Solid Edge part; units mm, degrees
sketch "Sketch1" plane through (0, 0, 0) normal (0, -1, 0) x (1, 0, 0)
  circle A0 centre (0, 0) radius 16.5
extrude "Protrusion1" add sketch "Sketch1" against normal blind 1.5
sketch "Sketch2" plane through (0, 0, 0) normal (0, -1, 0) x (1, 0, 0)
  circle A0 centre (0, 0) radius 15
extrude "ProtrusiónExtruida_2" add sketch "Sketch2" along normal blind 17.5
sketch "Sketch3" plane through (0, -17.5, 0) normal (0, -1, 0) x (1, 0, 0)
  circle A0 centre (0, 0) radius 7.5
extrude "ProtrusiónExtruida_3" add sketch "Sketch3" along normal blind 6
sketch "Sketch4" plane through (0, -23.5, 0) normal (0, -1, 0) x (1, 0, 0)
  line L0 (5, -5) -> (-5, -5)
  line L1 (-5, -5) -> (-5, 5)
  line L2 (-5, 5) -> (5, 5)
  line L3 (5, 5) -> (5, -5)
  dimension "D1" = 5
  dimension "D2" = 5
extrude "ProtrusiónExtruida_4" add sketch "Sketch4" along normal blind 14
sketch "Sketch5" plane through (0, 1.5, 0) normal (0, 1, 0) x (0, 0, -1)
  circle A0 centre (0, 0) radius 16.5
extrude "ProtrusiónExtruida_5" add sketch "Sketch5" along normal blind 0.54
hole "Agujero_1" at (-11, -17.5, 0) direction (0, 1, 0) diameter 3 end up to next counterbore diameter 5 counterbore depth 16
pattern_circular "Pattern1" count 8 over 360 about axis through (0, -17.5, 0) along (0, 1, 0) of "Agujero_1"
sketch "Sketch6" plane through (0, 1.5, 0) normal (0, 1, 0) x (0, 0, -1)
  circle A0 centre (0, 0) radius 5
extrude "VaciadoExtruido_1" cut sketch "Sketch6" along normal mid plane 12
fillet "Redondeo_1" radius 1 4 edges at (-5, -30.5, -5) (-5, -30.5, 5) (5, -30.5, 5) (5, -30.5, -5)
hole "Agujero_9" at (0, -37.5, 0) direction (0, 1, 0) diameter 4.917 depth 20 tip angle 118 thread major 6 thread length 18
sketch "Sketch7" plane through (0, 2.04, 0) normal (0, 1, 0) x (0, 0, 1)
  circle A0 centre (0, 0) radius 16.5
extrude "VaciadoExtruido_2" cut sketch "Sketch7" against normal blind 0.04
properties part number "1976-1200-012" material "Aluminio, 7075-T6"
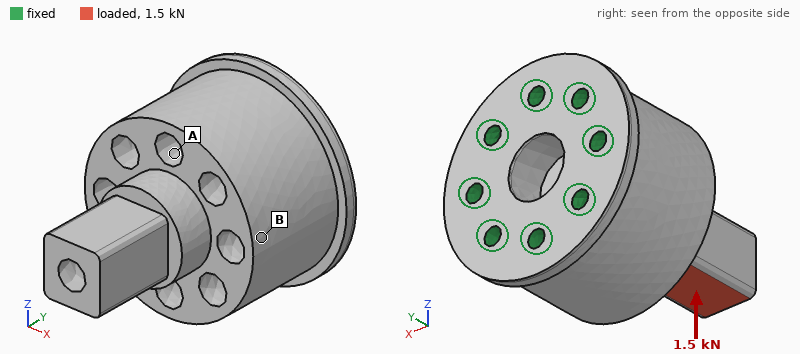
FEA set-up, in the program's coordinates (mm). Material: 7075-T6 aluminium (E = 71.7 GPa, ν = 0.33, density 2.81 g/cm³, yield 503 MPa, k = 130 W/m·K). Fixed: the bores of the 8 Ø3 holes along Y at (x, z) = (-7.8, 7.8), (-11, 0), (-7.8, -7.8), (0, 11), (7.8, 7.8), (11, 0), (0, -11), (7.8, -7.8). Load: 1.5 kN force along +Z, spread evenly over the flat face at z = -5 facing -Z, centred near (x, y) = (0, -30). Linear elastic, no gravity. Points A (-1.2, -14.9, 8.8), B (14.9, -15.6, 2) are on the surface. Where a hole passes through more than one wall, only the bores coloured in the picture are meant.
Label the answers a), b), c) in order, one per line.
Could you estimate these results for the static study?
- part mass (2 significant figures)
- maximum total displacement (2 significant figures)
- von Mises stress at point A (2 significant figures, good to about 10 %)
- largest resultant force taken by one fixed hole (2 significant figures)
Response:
a) 36 g
b) 58 µm
c) 33 MPa
d) 1000 N
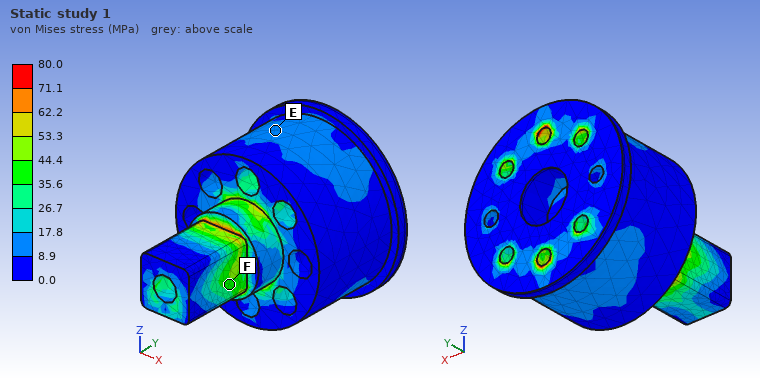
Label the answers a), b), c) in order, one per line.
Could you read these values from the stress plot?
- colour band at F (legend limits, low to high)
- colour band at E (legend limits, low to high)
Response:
a) 35.6 to 44.4 MPa
b) 8.9 to 17.8 MPa
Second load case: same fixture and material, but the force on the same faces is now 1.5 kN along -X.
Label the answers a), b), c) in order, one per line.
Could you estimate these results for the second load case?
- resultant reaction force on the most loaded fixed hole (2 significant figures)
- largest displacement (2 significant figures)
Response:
a) 1000 N
b) 66 µm
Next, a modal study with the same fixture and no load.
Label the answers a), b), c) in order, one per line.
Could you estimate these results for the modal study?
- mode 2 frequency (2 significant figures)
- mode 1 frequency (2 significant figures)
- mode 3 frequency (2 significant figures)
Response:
a) 15 kHz
b) 15 kHz
c) 29 kHz
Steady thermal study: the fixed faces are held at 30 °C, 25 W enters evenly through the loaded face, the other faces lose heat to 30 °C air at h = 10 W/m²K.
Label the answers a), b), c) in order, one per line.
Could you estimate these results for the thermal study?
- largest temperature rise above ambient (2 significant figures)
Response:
a) 42 K
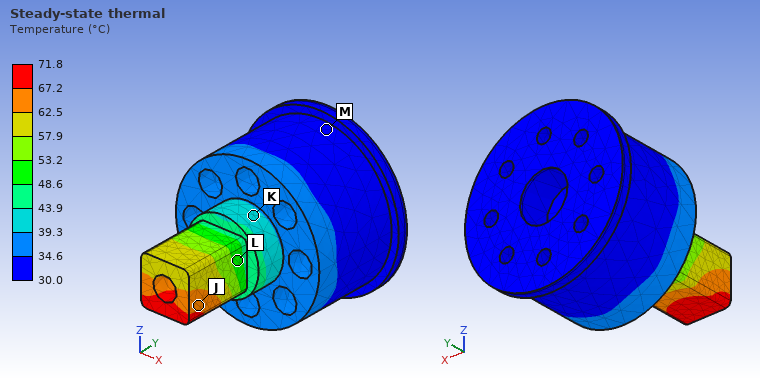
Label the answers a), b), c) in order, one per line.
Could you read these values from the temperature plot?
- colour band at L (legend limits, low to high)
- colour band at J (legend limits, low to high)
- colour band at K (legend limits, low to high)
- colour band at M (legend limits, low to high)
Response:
a) 48.6 to 53.2 °C
b) 62.5 to 67.2 °C
c) 39.3 to 43.9 °C
d) 30.0 to 34.6 °C
